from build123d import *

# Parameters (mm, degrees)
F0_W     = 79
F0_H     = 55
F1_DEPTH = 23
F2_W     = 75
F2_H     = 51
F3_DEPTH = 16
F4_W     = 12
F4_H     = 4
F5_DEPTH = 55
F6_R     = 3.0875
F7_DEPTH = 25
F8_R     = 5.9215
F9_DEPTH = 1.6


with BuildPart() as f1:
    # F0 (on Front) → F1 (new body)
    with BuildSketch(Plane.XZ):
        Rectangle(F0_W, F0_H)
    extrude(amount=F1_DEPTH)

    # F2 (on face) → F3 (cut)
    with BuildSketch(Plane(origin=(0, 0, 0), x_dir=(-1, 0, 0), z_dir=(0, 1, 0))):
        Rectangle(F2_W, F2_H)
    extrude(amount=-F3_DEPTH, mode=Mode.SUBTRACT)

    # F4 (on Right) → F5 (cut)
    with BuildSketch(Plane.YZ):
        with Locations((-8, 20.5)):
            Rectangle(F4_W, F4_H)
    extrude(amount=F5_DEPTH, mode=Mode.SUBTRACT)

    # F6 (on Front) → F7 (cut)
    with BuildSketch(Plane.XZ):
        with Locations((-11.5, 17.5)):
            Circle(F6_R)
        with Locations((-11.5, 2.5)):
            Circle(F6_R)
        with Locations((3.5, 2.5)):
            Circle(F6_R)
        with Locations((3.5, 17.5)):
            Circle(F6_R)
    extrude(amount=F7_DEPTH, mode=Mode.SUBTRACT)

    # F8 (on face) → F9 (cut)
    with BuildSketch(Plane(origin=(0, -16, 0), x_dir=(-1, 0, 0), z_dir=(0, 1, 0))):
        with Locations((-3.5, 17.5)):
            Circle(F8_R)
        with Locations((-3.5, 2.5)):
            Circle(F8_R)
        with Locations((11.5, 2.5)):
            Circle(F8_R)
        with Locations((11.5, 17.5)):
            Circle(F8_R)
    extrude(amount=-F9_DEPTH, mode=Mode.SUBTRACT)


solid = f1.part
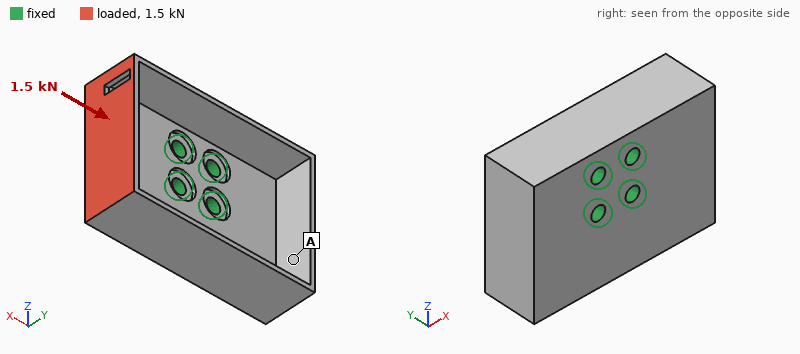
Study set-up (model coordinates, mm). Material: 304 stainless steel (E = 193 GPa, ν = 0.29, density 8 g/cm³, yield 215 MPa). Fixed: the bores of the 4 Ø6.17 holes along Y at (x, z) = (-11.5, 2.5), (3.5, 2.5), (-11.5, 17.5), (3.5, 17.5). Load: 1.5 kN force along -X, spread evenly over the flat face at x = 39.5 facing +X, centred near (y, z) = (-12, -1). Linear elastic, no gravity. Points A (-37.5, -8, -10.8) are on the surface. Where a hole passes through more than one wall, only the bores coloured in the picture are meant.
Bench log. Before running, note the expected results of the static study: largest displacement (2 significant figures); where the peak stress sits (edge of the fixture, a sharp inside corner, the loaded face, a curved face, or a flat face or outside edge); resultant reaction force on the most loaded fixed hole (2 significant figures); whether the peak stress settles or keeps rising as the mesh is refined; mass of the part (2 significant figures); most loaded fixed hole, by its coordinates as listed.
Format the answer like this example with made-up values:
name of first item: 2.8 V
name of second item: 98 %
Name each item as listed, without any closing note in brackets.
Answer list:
largest displacement: 76 µm
where the peak stress sits: a sharp inside corner
resultant reaction force on the most loaded fixed hole: 930 N
whether the peak stress settles or keeps rising as the mesh is refined: keeps rising
mass of the part: 300 g
most loaded fixed hole, by its coordinates as listed: (3.5, 2.5)
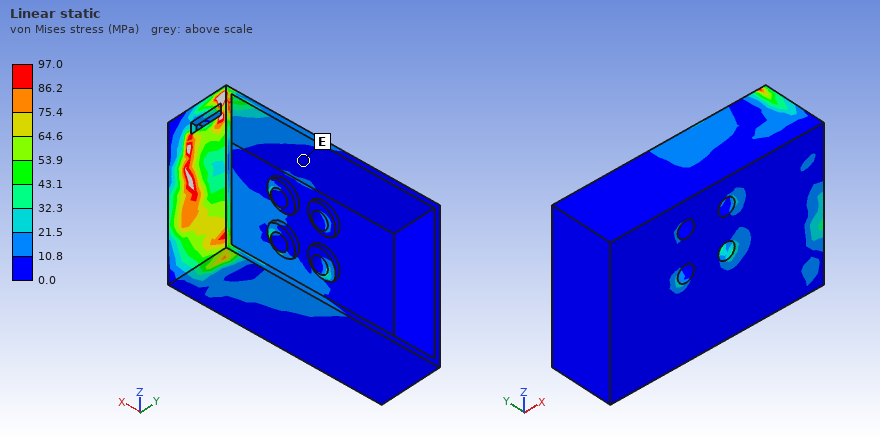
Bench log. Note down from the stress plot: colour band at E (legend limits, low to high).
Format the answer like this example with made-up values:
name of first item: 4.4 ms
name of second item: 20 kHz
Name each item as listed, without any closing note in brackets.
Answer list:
colour band at E: 0.0 to 10.8 MPa
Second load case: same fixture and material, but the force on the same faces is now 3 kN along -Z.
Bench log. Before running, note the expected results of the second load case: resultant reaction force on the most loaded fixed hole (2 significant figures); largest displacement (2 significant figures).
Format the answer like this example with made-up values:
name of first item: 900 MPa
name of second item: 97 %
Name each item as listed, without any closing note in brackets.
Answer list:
resultant reaction force on the most loaded fixed hole: 3.9 kN
largest displacement: 69 µm
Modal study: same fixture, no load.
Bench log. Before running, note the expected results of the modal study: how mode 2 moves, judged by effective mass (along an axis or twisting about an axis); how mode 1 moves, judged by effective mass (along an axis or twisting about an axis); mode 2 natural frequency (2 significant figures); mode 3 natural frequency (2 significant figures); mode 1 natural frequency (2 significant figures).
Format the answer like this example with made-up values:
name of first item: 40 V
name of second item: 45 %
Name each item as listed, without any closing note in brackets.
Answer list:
how mode 2 moves, judged by effective mass: along Y
how mode 1 moves, judged by effective mass: along Y
mode 2 natural frequency: 3600 Hz
mode 3 natural frequency: 5100 Hz
mode 1 natural frequency: 2900 Hz
